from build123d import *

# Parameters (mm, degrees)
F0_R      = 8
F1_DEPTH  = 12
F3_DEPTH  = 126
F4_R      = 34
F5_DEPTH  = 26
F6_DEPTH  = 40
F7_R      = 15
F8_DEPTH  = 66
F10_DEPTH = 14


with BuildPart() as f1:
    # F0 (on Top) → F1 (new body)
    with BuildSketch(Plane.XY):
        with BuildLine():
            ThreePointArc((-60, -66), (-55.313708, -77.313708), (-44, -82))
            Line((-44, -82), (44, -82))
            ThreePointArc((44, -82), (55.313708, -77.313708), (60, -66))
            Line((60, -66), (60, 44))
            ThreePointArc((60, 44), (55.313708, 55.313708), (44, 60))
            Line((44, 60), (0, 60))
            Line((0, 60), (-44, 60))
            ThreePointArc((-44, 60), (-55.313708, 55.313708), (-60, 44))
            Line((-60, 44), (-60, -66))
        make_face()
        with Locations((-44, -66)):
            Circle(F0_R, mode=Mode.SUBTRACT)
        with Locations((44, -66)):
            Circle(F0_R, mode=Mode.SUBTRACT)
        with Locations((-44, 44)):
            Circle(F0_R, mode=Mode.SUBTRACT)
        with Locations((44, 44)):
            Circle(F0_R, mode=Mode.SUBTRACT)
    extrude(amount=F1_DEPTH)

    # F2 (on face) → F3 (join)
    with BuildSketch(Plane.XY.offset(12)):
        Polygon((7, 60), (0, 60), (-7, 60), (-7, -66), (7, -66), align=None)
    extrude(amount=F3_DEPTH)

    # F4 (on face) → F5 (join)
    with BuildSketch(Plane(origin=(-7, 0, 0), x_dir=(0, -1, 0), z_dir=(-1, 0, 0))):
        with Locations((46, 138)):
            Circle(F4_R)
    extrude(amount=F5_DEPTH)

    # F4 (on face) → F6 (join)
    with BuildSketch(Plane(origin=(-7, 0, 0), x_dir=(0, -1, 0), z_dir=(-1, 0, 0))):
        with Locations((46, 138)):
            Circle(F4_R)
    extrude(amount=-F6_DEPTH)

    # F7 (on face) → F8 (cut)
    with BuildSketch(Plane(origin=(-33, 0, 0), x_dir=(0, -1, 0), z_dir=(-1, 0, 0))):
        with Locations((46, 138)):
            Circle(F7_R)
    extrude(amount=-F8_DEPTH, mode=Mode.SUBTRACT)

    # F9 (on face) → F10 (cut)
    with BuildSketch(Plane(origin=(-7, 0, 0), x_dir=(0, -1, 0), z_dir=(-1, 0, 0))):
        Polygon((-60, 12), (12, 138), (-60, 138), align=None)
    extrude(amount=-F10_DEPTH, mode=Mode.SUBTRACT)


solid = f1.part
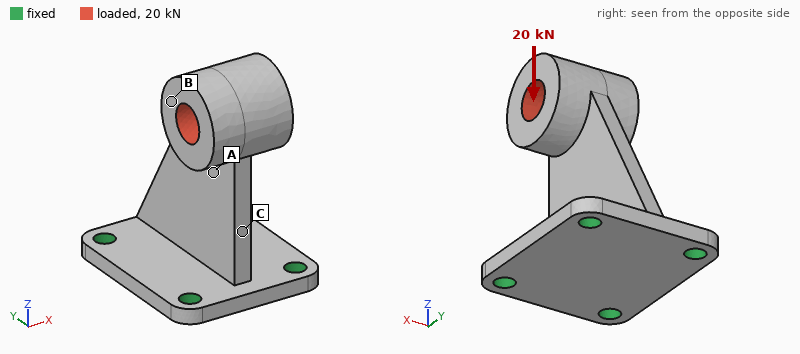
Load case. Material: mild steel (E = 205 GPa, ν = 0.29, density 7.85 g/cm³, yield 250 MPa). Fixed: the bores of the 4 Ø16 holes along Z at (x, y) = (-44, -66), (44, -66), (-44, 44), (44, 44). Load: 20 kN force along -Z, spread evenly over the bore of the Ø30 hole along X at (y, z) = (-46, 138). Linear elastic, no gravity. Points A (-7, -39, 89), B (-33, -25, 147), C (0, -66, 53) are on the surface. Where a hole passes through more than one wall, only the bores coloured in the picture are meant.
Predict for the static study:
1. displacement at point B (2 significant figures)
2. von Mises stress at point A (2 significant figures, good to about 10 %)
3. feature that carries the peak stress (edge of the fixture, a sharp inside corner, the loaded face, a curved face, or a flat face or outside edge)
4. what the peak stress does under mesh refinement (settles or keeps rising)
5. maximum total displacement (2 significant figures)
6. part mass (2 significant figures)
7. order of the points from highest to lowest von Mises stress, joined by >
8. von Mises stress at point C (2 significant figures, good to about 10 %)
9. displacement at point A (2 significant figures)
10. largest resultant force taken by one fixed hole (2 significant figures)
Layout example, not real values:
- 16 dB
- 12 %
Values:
- 72 µm
- 26 MPa
- edge of the fixture
- keeps rising
- 96 µm
- 4.1 kg
- C > A > B
- 44 MPa
- 50 µm
- 8.4 kN
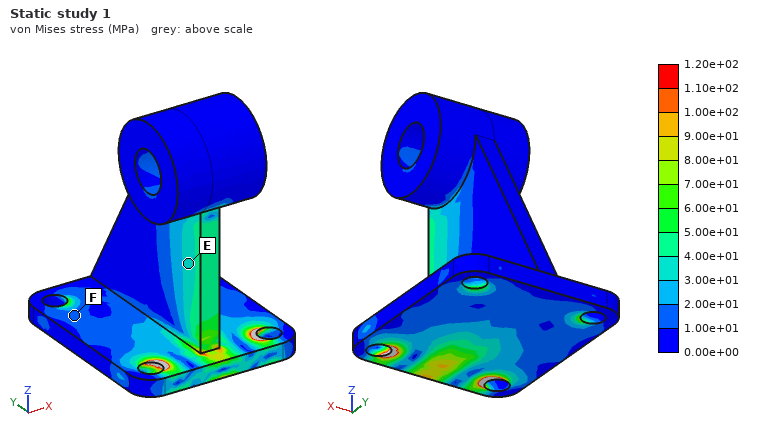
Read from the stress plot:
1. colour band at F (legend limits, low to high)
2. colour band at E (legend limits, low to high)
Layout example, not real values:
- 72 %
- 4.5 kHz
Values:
- 1.00e+01 to 2.00e+01 MPa
- 3.00e+01 to 4.00e+01 MPa
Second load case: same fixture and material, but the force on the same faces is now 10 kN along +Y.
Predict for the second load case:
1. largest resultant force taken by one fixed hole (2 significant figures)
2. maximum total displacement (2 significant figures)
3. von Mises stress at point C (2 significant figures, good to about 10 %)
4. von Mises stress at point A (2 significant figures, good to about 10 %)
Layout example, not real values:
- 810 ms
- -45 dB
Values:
- 6.9 kN
- 0.14 mm
- 39 MPa
- 16 MPa
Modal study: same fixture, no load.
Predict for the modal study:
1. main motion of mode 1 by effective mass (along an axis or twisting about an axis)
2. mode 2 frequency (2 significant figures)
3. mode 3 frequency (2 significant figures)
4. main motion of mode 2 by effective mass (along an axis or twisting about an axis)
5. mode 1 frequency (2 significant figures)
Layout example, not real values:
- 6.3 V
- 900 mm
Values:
- along X
- 1100 Hz
- 1200 Hz
- along Y
- 280 Hz
